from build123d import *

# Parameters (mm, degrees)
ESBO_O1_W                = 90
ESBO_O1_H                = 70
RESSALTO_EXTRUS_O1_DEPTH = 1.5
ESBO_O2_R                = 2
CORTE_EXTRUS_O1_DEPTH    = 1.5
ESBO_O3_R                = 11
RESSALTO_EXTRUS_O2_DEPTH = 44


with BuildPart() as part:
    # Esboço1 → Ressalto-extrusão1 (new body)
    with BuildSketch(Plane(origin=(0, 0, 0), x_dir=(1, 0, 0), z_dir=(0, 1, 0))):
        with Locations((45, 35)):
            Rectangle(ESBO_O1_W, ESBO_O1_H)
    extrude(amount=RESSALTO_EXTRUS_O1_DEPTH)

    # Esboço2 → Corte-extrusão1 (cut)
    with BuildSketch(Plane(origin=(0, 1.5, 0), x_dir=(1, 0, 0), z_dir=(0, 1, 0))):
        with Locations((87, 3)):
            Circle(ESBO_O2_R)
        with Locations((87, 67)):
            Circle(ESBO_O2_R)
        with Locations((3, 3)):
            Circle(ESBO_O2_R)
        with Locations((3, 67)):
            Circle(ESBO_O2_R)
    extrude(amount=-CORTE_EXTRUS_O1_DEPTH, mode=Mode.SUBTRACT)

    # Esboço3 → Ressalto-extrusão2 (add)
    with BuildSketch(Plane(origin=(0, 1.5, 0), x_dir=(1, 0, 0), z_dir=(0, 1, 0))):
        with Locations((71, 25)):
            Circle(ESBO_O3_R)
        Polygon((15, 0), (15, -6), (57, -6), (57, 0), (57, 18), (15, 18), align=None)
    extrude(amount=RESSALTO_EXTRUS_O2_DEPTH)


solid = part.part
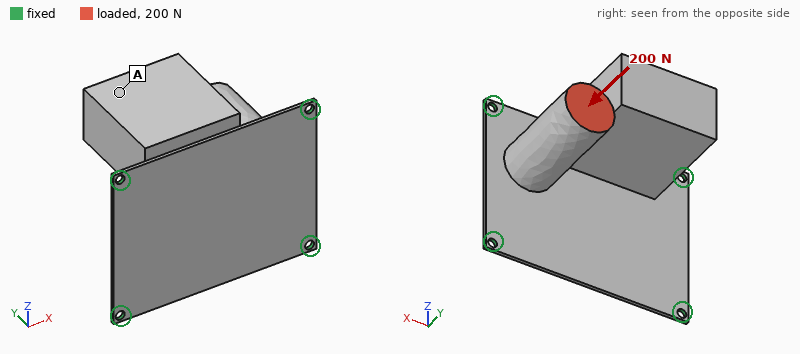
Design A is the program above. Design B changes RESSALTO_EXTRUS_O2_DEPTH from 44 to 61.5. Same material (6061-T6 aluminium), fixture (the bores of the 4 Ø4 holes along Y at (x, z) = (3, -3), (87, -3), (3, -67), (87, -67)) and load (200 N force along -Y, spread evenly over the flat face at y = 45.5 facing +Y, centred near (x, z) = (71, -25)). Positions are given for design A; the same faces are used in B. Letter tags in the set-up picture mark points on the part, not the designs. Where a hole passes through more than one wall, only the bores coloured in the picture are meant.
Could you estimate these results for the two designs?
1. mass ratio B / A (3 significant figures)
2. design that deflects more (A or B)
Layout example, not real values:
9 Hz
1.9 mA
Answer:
1.34
B
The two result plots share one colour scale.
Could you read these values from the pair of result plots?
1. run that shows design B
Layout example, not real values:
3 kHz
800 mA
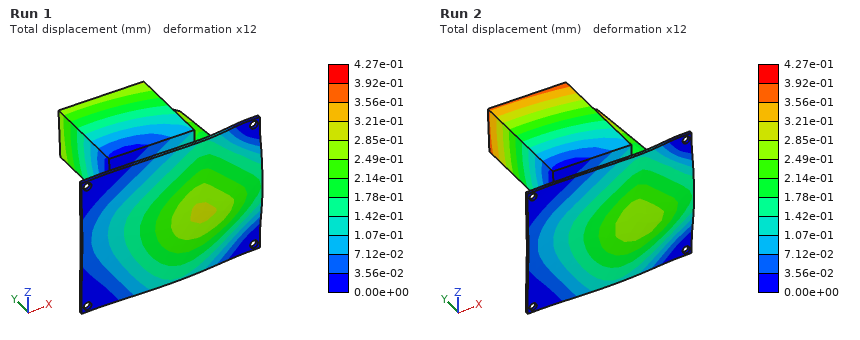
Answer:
Run 2
